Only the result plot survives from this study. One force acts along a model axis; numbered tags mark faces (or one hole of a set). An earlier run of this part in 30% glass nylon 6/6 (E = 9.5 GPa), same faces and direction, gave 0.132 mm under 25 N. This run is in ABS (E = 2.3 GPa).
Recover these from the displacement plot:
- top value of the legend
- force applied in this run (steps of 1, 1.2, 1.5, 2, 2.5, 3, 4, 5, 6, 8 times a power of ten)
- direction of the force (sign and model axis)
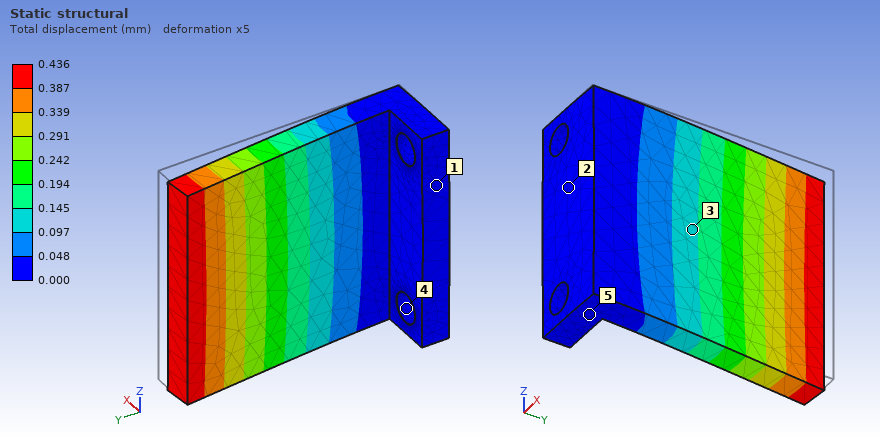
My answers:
0.436 mm
20 N
-X
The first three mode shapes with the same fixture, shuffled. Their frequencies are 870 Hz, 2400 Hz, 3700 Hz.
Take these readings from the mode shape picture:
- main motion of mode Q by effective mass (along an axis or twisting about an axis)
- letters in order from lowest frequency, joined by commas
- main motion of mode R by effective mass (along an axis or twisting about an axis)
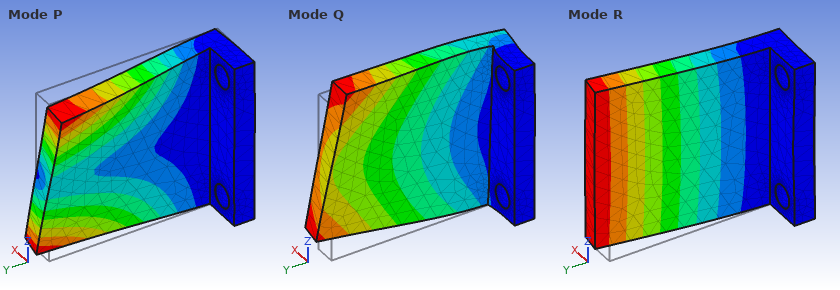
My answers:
along Z
R, P, Q
along X
